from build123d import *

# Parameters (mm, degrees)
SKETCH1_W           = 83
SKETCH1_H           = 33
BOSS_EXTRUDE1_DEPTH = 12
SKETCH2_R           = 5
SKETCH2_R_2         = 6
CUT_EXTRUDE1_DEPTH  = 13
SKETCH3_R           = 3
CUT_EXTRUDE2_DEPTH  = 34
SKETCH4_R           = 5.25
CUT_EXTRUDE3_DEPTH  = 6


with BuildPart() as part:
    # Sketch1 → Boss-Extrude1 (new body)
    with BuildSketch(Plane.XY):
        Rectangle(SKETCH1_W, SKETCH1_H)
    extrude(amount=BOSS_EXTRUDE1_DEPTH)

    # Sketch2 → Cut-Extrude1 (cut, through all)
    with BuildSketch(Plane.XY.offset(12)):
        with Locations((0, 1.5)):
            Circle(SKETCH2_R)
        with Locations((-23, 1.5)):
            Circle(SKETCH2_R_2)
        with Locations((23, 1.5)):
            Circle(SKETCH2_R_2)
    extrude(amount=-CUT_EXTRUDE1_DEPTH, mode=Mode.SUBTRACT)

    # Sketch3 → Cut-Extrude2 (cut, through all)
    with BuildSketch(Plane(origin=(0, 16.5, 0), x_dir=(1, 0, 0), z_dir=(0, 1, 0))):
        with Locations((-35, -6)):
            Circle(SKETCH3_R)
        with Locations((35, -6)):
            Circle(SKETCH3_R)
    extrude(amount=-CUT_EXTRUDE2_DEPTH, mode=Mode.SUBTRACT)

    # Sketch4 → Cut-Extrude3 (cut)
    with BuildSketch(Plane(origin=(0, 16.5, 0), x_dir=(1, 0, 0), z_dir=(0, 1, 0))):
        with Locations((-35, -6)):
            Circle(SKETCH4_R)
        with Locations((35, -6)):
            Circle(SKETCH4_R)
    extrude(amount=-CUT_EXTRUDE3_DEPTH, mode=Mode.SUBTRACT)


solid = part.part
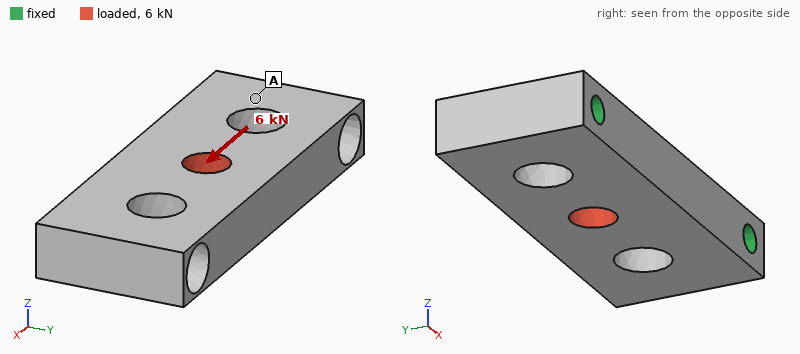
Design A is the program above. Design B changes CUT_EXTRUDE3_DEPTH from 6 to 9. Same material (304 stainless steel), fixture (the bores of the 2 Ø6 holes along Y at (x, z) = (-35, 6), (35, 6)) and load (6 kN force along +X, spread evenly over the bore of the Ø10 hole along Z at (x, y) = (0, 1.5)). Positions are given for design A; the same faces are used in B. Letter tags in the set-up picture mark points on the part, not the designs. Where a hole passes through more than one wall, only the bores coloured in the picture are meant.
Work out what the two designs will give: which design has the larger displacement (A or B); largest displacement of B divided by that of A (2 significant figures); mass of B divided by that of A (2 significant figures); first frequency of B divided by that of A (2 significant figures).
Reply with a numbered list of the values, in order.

1. B
2. 1.2
3. 0.99
4. 0.93
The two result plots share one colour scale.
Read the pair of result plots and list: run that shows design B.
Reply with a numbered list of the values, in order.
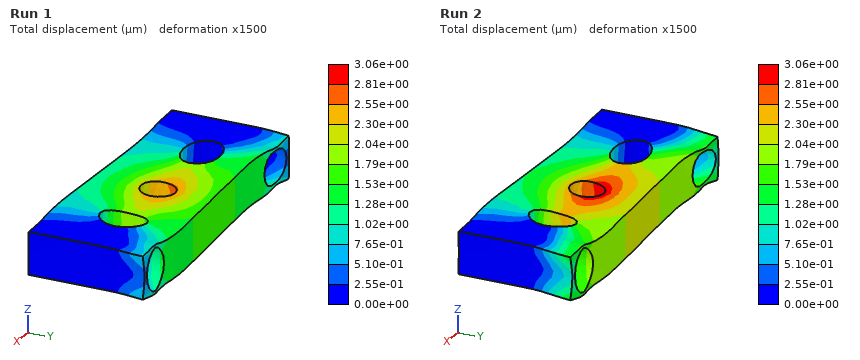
1. Run 2
